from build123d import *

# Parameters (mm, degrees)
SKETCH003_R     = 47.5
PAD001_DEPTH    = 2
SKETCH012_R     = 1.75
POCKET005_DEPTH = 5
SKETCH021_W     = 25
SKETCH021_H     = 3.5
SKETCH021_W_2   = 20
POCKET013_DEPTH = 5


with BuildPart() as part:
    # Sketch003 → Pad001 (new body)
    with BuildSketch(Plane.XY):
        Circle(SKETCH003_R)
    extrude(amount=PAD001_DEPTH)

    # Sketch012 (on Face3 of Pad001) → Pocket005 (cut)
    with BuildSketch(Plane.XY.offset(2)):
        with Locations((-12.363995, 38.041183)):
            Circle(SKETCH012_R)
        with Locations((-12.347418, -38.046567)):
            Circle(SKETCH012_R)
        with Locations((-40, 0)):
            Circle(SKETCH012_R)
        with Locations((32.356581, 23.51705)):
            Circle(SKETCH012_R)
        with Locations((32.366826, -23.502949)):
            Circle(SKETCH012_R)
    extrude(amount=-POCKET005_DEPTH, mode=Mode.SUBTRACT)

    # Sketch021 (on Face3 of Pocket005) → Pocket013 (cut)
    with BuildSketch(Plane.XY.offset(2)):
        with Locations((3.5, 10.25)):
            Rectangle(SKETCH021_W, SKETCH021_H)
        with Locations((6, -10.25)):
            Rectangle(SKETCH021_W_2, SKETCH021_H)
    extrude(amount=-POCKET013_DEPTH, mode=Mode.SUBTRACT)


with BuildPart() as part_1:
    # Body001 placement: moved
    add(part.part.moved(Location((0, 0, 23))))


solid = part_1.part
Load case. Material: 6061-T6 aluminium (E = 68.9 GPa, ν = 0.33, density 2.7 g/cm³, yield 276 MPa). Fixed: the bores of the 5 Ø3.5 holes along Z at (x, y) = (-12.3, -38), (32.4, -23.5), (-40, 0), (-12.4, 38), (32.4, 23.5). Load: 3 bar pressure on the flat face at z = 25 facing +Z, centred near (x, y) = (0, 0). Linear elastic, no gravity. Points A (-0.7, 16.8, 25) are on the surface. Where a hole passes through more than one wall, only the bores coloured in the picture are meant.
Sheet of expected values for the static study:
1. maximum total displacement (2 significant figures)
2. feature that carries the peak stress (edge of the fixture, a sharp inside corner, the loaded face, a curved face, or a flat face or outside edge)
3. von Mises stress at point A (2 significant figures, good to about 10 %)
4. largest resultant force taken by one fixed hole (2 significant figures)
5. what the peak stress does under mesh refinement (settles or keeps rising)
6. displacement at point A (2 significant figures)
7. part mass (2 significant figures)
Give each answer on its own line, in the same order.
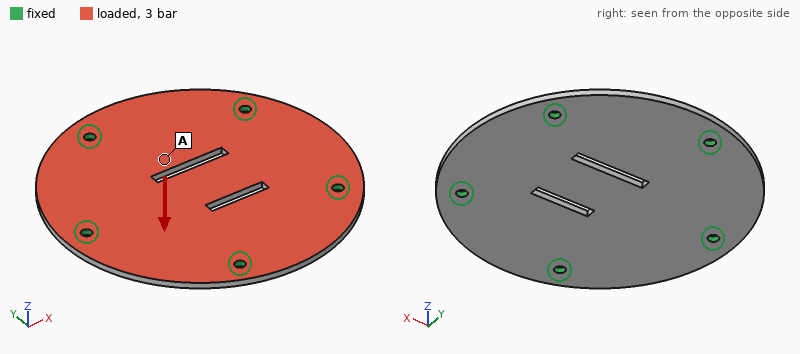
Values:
0.37 mm
edge of the fixture
39 MPa
420 N
keeps rising
0.26 mm
37 g
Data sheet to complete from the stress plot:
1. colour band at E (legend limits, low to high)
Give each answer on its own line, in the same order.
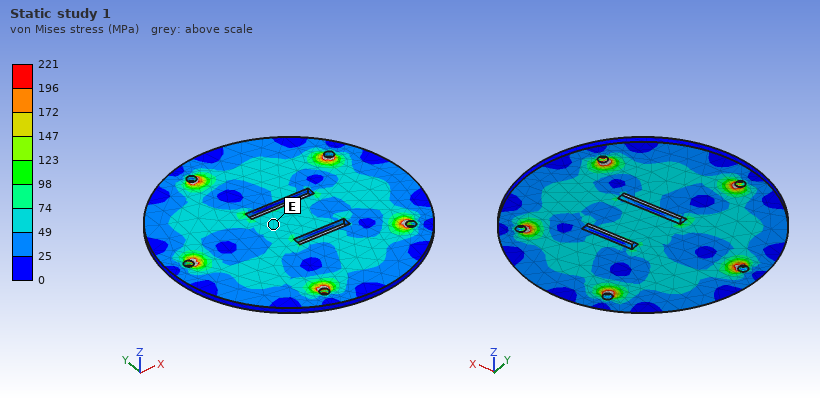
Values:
49 to 74 MPa
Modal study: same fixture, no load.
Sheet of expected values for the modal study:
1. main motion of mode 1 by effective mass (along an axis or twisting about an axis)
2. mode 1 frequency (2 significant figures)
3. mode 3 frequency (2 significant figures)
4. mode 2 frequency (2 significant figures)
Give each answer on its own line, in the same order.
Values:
along Z
2400 Hz
4000 Hz
4000 Hz
